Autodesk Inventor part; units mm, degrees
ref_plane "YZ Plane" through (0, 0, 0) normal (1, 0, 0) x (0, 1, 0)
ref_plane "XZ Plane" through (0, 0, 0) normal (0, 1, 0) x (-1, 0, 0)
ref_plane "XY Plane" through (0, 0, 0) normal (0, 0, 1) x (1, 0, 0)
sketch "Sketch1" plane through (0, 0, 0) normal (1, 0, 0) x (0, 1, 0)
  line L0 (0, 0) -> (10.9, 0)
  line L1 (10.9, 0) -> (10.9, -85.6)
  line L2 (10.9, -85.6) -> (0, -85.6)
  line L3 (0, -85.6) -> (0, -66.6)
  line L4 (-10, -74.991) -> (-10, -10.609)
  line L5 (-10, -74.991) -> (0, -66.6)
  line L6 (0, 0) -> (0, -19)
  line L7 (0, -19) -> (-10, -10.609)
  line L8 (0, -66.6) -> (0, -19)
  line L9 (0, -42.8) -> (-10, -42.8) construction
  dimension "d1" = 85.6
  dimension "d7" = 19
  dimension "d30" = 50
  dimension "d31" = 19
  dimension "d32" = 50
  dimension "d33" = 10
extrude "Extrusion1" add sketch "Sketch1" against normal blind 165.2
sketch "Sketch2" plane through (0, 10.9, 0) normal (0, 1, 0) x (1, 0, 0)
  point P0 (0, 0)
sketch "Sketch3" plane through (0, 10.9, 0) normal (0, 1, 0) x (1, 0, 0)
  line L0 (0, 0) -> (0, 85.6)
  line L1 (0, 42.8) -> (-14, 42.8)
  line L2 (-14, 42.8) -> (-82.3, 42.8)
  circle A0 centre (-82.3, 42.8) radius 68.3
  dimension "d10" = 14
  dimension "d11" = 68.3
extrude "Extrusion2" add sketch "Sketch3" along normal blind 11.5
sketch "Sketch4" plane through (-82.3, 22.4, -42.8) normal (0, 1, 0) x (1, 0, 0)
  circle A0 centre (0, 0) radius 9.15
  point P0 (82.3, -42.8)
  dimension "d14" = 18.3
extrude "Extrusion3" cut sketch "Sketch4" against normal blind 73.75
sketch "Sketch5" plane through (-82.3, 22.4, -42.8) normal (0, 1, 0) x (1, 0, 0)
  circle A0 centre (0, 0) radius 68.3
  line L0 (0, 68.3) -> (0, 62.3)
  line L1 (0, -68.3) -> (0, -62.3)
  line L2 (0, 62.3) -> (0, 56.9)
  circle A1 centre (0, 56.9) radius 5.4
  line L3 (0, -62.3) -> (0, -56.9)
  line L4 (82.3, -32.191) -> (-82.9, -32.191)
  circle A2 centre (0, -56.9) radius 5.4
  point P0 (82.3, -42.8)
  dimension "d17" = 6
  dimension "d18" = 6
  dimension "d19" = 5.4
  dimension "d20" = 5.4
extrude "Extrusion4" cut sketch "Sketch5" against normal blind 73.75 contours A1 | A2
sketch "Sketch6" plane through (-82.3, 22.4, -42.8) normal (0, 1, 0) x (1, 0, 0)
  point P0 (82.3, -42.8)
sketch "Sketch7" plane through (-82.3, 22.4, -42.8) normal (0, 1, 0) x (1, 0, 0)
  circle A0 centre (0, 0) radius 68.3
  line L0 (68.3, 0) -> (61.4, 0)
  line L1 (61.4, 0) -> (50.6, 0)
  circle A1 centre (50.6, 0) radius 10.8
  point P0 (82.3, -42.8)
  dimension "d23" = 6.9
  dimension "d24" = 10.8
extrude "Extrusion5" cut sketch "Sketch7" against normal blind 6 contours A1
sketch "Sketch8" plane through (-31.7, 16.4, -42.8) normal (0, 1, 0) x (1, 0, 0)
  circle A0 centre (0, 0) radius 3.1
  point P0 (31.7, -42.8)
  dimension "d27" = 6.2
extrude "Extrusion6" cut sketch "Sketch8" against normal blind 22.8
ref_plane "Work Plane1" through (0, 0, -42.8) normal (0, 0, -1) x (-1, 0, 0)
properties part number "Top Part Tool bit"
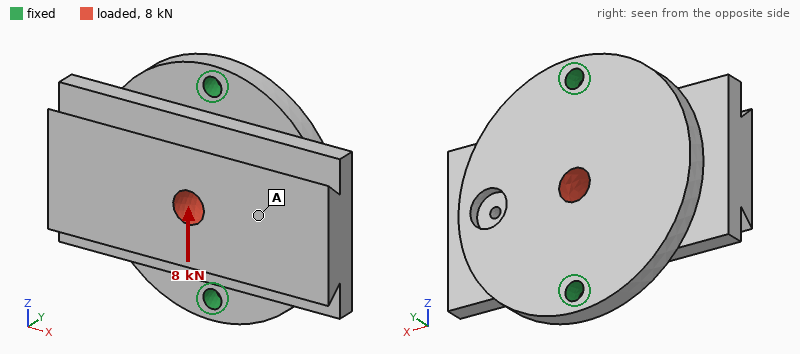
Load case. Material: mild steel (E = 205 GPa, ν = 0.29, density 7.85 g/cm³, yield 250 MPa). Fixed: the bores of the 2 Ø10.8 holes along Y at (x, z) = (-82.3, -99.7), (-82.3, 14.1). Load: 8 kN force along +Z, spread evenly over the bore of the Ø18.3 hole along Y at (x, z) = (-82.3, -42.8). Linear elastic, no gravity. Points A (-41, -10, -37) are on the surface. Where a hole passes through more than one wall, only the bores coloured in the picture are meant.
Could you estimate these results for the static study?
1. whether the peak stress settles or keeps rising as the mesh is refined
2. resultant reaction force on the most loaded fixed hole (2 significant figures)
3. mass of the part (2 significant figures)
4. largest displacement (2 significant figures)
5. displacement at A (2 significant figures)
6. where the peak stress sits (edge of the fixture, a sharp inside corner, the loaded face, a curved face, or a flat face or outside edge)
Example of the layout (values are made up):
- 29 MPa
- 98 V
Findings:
- keeps rising
- 4.1 kN
- 3.2 kg
- 2.2 µm
- 1.5 µm
- edge of the fixture
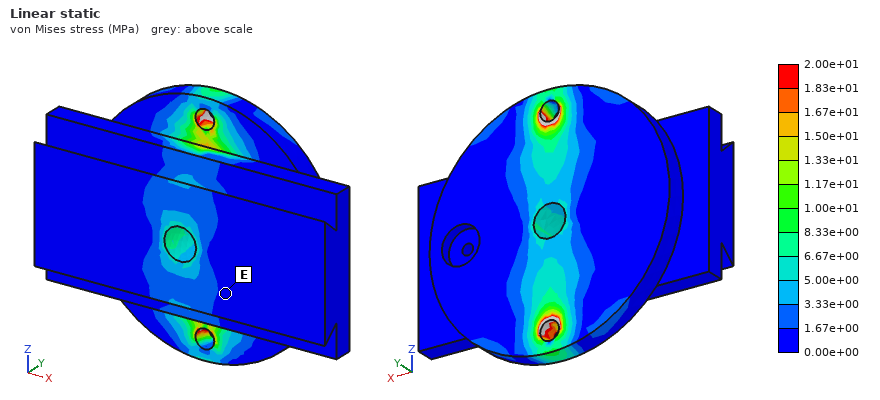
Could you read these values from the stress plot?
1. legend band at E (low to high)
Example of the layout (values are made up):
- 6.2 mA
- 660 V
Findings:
- 0.00e+00 to 1.67e+00 MPa
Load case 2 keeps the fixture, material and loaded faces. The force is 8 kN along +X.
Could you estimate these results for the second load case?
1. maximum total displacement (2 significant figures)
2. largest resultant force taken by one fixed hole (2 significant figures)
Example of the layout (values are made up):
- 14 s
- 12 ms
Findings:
- 30 µm
- 4.0 kN
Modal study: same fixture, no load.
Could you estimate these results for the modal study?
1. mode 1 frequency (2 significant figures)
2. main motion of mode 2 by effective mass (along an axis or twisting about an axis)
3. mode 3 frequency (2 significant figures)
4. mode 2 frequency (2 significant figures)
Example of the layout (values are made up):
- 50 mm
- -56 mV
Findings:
- 1000 Hz
- along Y
- 5500 Hz
- 2700 Hz
